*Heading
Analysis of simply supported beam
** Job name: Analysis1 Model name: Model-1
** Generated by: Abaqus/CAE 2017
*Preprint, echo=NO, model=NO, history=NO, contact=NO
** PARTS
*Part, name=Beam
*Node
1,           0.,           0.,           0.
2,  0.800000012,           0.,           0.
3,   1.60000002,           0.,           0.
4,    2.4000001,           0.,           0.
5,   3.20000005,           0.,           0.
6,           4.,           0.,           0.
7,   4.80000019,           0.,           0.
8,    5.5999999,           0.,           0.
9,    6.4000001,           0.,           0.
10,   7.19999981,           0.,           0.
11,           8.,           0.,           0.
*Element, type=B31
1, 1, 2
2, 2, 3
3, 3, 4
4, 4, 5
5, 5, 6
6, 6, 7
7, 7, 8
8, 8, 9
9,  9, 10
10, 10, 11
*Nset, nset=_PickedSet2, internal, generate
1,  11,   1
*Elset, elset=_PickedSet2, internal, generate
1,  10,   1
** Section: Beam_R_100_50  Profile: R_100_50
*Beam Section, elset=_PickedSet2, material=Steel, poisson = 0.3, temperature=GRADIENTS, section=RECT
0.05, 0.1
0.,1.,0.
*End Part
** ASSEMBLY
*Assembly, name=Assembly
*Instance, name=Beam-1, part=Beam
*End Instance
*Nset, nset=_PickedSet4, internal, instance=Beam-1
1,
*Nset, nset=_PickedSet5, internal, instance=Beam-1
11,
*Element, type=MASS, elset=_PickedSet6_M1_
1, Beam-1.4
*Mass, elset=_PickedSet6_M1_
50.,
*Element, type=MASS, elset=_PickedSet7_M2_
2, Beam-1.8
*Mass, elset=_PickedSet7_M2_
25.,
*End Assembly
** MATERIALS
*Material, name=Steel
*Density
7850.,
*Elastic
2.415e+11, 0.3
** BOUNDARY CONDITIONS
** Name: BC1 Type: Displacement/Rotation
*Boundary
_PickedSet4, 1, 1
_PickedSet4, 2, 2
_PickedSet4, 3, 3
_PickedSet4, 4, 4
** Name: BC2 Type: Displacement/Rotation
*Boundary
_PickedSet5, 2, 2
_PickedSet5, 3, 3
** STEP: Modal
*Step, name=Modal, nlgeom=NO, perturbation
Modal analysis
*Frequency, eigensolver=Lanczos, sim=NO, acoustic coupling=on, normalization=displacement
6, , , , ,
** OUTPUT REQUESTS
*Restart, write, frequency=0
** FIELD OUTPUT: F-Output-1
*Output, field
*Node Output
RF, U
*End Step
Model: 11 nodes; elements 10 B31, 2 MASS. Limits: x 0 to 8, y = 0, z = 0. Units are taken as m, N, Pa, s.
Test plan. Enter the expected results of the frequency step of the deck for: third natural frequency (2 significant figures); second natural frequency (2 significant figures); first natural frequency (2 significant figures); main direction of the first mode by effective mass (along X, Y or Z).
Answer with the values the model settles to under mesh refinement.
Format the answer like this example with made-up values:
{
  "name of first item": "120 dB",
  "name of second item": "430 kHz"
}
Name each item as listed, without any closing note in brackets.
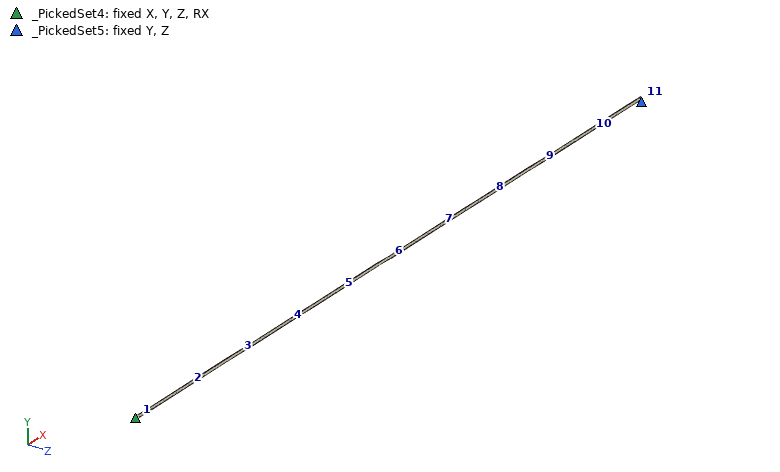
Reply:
{
  "third natural frequency": "6.6 Hz",
  "second natural frequency": "3.4 Hz",
  "first natural frequency": "1.7 Hz",
  "main direction of the first mode by effective mass": "along Y"
}
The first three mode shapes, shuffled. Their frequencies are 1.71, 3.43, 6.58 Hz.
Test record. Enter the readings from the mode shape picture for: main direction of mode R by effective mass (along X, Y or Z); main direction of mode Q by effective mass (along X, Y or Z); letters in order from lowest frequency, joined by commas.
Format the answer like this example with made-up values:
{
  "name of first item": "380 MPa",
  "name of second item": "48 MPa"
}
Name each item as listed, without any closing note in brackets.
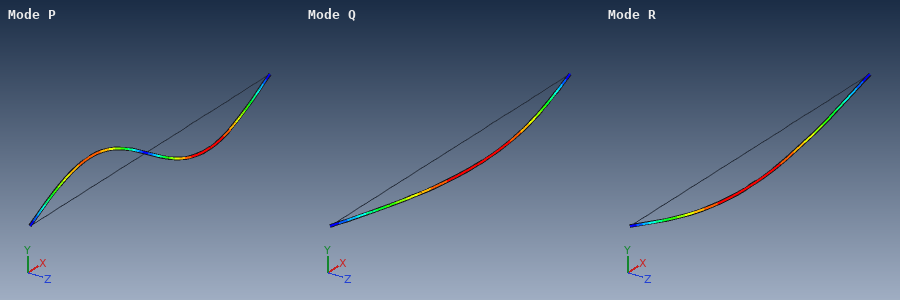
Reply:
{
  "main direction of mode R by effective mass": "along Y",
  "main direction of mode Q by effective mass": "along Z",
  "letters in order from lowest frequency, joined by commas": "R, Q, P"
}
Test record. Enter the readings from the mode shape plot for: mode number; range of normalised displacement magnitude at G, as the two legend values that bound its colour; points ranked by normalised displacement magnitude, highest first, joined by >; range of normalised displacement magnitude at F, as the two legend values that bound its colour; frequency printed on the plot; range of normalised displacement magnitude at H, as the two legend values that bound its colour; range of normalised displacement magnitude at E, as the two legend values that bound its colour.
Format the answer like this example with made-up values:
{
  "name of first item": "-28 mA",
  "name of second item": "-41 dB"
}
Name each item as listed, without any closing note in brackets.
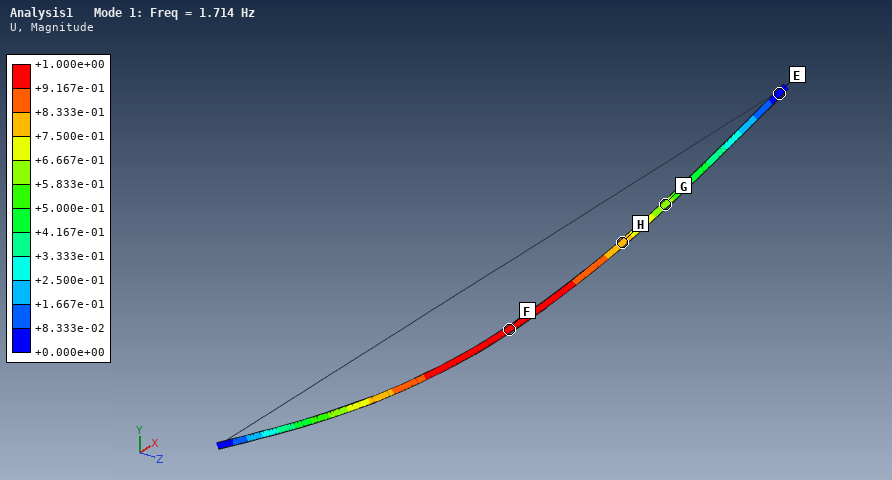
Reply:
{
  "mode number": "1",
  "range of normalised displacement magnitude at G, as the two legend values that bound its colour": "+5.833e-01 to +6.667e-01",
  "points ranked by normalised displacement magnitude, highest first, joined by >": "F > H > G > E",
  "range of normalised displacement magnitude at F, as the two legend values that bound its colour": "+9.167e-01 to +1.000e+00",
  "frequency printed on the plot": "1.714 Hz",
  "range of normalised displacement magnitude at H, as the two legend values that bound its colour": "+7.500e-01 to +8.333e-01",
  "range of normalised displacement magnitude at E, as the two legend values that bound its colour": "+0.000e+00 to +8.333e-02"
}
